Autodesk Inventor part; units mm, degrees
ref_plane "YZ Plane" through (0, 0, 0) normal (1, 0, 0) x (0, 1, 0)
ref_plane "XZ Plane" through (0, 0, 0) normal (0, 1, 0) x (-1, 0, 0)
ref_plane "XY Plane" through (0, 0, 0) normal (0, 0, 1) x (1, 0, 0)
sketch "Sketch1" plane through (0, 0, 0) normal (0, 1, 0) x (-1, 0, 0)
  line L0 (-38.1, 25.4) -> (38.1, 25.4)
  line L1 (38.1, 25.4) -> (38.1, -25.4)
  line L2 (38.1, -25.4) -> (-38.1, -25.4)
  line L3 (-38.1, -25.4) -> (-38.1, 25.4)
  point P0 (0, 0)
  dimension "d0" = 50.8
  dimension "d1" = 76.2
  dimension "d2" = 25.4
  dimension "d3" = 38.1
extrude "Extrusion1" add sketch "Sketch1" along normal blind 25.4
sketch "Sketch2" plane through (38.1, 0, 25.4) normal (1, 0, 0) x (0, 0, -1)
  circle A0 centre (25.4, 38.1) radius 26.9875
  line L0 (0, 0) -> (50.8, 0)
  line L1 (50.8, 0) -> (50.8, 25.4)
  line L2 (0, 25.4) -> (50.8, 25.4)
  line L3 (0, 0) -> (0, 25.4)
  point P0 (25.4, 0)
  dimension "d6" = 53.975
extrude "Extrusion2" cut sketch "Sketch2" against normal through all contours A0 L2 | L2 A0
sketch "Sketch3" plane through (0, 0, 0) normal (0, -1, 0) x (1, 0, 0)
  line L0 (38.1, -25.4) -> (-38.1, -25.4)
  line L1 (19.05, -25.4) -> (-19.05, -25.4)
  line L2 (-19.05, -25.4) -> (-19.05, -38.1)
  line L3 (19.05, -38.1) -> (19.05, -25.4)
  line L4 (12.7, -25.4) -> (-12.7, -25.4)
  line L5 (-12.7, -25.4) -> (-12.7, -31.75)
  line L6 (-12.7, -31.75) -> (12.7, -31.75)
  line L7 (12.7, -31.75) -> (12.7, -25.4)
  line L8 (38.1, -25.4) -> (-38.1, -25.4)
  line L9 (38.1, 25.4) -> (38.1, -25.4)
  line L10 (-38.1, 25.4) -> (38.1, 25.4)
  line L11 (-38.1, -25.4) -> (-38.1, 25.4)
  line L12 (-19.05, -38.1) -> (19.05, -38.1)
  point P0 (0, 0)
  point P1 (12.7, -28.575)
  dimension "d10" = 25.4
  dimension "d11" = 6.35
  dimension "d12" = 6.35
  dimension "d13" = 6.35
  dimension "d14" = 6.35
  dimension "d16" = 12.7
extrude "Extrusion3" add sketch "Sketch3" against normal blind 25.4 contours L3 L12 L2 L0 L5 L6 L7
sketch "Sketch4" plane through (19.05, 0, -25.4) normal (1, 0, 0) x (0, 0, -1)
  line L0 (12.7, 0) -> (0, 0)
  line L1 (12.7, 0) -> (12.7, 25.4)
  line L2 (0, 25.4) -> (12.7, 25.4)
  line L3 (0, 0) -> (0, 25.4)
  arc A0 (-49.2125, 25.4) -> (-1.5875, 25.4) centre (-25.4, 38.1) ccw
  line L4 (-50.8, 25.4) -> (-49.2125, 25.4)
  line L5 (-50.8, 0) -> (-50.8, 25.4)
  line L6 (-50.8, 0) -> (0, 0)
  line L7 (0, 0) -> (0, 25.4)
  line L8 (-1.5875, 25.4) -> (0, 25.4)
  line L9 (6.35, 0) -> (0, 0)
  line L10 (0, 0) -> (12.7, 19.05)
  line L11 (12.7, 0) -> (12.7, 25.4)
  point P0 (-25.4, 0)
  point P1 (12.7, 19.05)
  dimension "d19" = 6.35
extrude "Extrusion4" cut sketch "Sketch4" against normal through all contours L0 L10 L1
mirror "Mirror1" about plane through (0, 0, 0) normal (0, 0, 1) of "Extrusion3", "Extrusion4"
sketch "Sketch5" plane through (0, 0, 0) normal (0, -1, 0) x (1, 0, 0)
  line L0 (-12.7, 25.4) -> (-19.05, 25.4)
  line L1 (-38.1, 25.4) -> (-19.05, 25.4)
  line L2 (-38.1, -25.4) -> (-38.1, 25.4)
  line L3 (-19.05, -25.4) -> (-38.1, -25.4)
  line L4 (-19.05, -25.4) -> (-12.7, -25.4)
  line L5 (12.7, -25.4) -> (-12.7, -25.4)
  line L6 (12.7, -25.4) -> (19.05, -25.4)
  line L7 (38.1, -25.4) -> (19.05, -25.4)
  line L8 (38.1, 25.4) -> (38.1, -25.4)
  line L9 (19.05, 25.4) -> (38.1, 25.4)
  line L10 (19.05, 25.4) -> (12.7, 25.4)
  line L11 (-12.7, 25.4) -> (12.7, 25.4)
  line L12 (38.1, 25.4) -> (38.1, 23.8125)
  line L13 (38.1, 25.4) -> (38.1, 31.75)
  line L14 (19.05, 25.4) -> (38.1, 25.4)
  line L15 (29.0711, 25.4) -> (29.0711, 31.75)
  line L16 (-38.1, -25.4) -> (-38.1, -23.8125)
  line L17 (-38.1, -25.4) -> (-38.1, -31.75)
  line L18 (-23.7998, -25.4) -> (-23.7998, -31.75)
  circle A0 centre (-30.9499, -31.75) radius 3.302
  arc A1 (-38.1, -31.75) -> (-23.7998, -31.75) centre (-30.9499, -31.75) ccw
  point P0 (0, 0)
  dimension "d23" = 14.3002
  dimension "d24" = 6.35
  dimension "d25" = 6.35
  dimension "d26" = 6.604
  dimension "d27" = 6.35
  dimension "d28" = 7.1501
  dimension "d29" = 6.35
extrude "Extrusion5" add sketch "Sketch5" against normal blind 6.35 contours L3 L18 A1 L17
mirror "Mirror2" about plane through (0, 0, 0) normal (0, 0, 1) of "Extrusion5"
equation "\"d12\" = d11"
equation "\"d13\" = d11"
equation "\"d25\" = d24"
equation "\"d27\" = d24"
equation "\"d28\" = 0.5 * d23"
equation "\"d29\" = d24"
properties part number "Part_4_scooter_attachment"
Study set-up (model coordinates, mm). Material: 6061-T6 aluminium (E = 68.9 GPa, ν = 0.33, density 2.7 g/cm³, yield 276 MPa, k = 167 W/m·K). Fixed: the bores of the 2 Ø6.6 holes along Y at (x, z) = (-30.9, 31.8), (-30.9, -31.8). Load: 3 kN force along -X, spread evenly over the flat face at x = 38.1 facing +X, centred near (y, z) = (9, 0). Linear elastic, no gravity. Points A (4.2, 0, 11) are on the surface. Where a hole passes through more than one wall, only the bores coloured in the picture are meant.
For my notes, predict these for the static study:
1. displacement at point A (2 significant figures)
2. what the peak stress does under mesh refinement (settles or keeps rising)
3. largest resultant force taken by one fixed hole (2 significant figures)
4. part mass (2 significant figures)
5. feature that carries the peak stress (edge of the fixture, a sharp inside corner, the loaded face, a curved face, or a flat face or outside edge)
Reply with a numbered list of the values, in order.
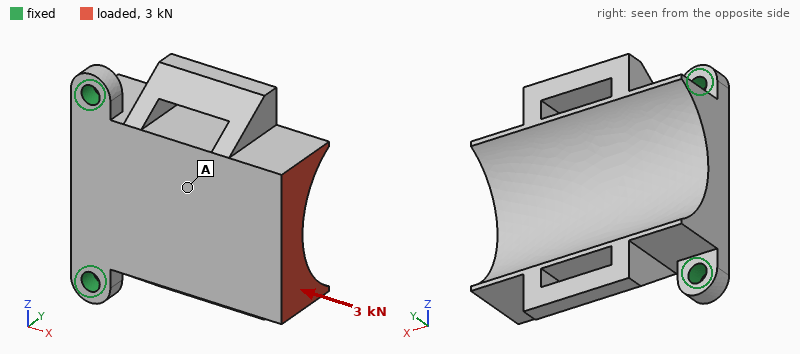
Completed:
1. 0.065 mm
2. keeps rising
3. 1.6 kN
4. 190 g
5. edge of the fixture
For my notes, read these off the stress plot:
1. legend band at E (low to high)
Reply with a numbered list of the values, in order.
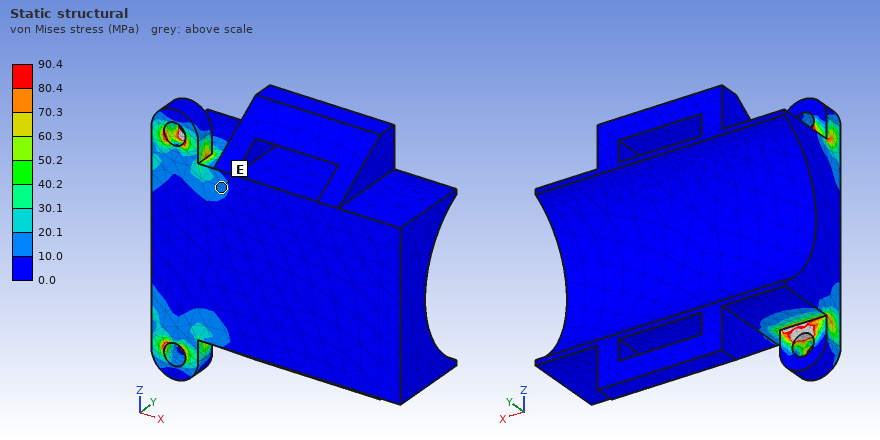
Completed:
1. 10.0 to 20.1 MPa
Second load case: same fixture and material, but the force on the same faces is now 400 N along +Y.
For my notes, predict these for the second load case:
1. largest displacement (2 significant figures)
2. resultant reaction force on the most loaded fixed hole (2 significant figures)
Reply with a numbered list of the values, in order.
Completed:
1. 0.26 mm
2. 290 N
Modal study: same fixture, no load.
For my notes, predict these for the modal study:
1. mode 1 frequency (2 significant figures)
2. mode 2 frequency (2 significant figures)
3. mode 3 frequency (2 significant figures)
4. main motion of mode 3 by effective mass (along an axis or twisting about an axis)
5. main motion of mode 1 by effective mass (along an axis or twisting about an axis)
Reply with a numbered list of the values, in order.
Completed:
1. 850 Hz
2. 3900 Hz
3. 4000 Hz
4. along Z
5. along Y
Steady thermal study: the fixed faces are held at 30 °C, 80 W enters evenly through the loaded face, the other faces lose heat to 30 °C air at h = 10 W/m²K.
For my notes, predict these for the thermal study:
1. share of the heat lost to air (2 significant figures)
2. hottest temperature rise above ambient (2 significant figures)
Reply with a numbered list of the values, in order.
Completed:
1. 7.6 %
2. 58 K
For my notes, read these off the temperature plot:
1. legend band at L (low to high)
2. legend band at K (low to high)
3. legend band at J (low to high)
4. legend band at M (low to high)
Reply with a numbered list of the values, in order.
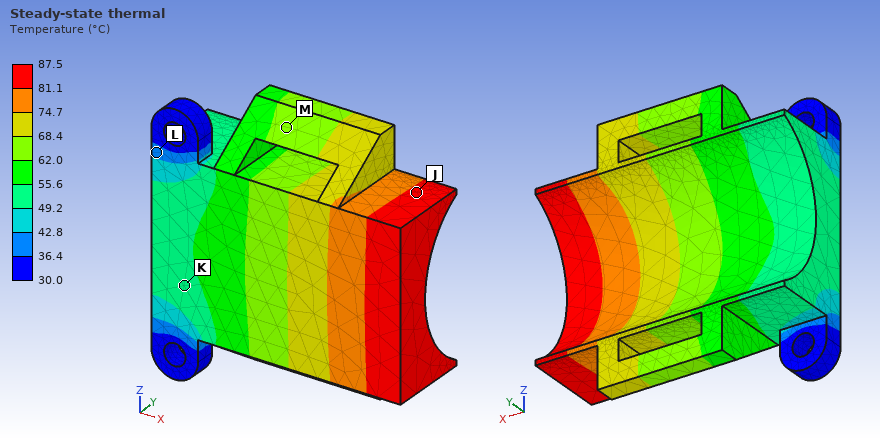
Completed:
1. 36.4 to 42.8 °C
2. 49.2 to 55.6 °C
3. 81.1 to 87.5 °C
4. 62.0 to 68.4 °C
